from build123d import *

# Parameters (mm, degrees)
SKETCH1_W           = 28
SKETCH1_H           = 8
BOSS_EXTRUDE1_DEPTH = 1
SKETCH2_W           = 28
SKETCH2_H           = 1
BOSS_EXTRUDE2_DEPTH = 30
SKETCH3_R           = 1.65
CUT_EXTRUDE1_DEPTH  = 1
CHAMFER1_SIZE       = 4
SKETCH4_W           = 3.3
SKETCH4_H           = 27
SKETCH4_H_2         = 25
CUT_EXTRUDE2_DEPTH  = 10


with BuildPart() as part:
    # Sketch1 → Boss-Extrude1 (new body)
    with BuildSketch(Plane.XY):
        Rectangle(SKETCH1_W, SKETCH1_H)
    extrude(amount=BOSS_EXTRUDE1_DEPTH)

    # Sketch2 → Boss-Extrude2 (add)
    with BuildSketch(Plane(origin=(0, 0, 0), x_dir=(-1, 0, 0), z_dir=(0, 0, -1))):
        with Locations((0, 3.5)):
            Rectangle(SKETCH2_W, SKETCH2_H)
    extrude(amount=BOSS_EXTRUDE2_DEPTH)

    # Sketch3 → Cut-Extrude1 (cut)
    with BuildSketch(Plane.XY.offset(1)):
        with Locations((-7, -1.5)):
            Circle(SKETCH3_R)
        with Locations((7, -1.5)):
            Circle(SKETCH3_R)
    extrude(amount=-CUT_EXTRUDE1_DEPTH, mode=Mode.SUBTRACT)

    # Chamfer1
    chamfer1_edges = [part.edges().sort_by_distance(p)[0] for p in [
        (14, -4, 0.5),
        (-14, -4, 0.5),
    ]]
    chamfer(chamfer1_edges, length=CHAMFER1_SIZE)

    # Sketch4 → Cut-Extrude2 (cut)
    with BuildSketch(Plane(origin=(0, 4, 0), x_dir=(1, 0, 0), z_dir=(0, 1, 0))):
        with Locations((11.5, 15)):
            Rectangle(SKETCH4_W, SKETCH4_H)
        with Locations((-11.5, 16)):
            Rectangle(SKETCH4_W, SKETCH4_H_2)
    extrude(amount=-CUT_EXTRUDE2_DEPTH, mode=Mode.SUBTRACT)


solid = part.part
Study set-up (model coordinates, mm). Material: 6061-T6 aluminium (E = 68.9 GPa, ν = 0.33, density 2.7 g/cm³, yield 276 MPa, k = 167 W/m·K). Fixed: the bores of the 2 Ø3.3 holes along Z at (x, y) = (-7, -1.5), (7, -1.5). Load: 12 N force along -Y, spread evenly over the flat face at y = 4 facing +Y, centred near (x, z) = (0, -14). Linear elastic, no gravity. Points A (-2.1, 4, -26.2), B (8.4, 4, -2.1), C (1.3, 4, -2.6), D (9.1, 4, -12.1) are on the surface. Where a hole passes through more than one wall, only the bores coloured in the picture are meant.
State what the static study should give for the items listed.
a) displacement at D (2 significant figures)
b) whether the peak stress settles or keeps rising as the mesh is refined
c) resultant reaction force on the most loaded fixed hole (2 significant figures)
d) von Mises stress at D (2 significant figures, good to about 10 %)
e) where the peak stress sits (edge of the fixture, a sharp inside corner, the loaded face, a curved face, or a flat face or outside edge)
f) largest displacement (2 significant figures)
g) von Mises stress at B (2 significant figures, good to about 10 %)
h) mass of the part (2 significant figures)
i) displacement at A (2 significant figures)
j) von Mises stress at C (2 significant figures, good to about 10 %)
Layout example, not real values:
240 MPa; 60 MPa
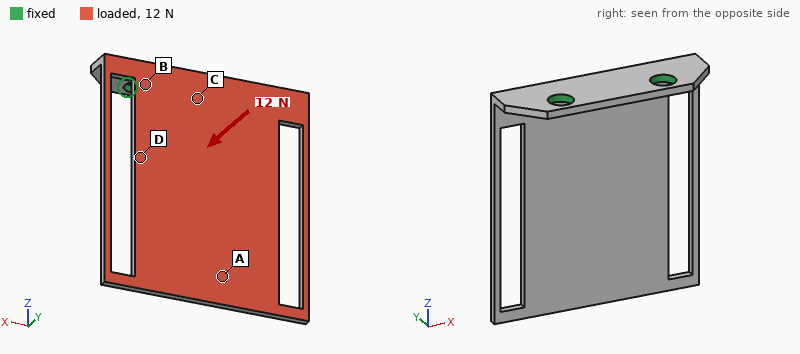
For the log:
0.13 mm; keeps rising; 6.4 N; 18 MPa; edge of the fixture; 0.44 mm; 40 MPa; 2.3 g; 0.37 mm; 34 MPa
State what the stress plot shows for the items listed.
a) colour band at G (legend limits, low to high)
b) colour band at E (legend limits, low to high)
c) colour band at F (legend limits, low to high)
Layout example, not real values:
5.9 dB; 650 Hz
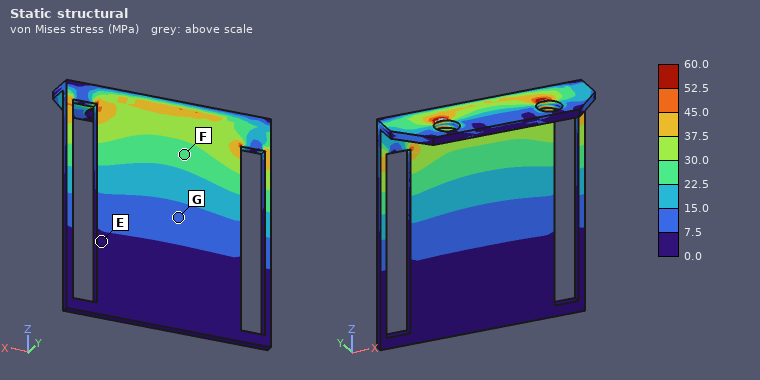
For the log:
7.5 to 15.0 MPa; 0.0 to 7.5 MPa; 22.5 to 30.0 MPa
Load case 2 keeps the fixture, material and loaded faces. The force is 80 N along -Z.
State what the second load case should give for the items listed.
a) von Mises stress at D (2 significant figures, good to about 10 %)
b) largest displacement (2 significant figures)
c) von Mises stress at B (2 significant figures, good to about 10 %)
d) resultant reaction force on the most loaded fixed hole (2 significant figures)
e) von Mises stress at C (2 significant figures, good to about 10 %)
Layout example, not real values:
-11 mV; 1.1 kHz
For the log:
8.7 MPa; 0.26 mm; 14 MPa; 41 N; 11 MPa
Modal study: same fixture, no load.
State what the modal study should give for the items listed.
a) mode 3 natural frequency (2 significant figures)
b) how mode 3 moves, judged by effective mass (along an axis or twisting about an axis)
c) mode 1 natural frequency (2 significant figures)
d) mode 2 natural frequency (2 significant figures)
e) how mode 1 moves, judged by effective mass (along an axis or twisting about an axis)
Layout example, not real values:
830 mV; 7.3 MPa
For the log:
4000 Hz; along X; 750 Hz; 2300 Hz; along Y
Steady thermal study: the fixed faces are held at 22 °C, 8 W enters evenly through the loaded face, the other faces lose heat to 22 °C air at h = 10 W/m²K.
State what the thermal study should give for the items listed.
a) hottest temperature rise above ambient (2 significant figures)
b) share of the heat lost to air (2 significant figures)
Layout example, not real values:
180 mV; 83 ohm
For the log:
40 K; 3.4 %
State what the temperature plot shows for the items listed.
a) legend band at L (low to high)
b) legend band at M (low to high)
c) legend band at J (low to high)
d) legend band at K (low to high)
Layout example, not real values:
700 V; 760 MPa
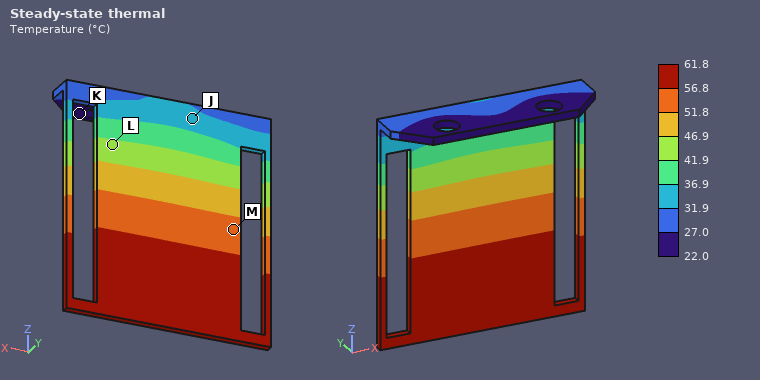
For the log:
41.9 to 46.9 °C; 51.8 to 56.8 °C; 31.9 to 36.9 °C; 22.0 to 27.0 °C
